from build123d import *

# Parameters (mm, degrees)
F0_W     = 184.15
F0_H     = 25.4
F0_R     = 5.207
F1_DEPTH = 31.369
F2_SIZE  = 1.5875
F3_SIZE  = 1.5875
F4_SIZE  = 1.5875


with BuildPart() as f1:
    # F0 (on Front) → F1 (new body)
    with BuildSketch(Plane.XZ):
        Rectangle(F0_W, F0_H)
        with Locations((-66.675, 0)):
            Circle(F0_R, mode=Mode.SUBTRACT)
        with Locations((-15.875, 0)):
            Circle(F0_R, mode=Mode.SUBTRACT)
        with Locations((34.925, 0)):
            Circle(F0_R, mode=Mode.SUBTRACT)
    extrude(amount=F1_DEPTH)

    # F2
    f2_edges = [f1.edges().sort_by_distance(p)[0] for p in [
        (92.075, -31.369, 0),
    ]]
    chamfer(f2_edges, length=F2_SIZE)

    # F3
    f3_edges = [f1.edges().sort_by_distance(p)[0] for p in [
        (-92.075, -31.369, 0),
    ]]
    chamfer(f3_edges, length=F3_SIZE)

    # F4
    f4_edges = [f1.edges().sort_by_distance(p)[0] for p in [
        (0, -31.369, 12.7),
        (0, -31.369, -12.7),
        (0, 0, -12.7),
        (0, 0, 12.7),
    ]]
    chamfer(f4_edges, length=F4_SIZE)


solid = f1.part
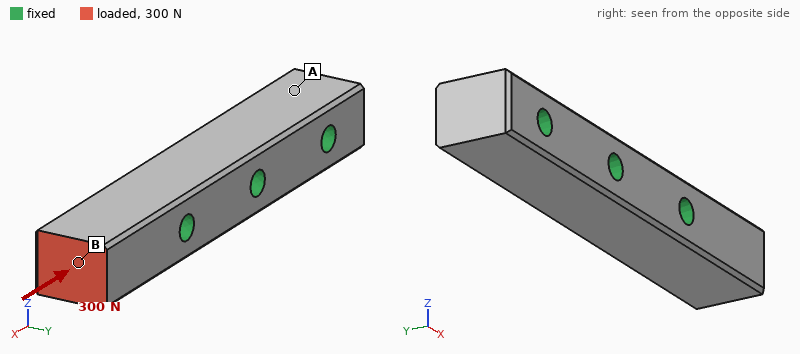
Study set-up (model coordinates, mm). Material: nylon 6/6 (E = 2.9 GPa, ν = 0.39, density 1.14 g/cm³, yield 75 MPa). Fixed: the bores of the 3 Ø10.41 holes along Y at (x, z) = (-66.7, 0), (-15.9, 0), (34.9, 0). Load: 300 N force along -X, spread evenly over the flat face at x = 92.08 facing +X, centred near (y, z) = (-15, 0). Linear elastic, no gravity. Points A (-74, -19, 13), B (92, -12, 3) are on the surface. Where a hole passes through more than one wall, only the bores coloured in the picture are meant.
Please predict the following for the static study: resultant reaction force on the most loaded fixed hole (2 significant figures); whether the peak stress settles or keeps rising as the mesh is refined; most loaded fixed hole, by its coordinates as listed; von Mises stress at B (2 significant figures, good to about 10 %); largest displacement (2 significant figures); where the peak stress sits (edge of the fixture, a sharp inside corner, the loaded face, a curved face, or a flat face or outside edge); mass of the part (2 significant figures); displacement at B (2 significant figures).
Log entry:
290 N
keeps rising
(34.9, 0)
0.38 MPa
8.6 µm
edge of the fixture
160 g
7.8 µm
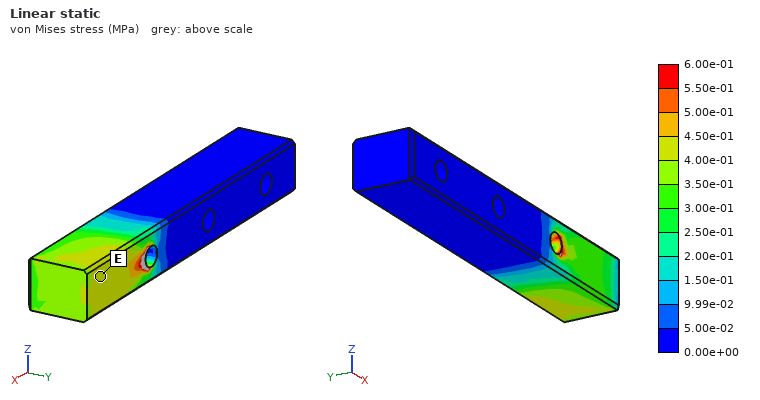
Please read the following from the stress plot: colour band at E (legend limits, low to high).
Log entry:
4.00e-01 to 4.50e-01 MPa
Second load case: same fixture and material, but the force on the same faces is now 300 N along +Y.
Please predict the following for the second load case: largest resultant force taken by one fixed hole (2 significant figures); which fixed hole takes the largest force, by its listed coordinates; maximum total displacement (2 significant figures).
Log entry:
320 N
(34.9, 0)
0.12 mm
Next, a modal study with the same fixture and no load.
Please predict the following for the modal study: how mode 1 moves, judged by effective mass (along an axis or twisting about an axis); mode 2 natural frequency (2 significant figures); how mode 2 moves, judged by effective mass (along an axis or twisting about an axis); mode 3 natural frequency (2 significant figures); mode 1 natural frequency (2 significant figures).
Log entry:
along Z
2200 Hz
along Y
4000 Hz
1600 Hz
